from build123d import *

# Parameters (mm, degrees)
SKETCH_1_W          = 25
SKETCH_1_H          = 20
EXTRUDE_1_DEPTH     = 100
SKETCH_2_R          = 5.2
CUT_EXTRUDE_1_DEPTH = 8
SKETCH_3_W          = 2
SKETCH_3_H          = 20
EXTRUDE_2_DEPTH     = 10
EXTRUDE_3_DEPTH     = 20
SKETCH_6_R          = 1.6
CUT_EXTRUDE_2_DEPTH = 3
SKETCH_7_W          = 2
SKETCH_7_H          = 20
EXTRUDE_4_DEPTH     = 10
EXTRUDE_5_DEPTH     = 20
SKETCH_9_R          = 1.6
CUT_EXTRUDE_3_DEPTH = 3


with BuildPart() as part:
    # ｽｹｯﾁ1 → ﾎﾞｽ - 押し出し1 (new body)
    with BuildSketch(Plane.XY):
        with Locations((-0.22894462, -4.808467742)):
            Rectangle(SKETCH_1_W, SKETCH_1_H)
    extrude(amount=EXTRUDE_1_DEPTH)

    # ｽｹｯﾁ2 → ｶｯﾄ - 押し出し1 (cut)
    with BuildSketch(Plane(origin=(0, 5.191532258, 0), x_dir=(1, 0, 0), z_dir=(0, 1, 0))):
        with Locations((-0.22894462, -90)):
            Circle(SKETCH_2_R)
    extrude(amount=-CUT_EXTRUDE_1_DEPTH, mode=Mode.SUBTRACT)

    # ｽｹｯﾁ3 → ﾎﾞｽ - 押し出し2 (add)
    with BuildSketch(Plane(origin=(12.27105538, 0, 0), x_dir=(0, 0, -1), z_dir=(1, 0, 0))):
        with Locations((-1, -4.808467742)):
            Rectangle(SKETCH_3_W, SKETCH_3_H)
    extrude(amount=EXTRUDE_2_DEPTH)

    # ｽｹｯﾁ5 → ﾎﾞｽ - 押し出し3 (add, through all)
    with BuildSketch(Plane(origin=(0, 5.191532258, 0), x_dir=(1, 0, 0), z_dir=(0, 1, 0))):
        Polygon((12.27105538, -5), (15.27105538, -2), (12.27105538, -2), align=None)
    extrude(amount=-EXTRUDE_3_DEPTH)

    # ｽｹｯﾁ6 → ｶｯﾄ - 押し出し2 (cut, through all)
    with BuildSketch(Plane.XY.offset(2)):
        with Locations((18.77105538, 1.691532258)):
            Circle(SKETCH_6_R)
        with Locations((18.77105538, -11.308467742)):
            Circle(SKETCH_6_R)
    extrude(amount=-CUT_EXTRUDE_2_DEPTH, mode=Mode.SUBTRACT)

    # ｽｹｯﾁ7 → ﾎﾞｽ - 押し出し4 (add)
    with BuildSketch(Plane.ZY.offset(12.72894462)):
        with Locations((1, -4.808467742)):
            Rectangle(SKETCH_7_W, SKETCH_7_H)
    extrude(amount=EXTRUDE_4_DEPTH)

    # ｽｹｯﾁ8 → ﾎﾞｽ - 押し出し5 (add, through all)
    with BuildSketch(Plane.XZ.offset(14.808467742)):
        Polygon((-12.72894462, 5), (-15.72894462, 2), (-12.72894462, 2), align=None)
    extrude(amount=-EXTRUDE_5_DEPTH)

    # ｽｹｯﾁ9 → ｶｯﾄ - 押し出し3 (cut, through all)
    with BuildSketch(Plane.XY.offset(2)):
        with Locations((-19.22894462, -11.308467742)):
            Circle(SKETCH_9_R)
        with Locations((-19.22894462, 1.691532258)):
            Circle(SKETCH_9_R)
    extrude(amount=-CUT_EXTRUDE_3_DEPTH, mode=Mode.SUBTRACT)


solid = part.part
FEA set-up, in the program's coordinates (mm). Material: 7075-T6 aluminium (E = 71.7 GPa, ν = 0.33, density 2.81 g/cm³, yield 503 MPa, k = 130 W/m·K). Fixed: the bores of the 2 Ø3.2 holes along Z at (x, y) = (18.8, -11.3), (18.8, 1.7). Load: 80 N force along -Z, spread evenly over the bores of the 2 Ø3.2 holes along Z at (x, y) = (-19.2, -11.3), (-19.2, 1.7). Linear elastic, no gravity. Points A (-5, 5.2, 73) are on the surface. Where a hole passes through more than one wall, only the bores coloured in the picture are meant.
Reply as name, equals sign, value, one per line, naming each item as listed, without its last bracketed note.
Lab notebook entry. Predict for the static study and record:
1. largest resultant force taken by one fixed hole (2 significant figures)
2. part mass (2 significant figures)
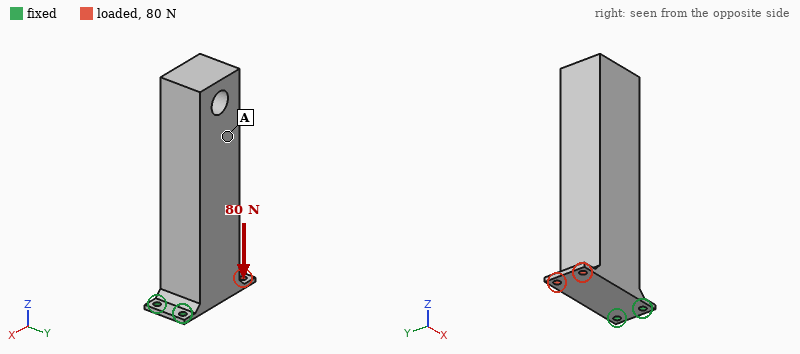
largest resultant force taken by one fixed hole = 41 N
part mass = 140 g
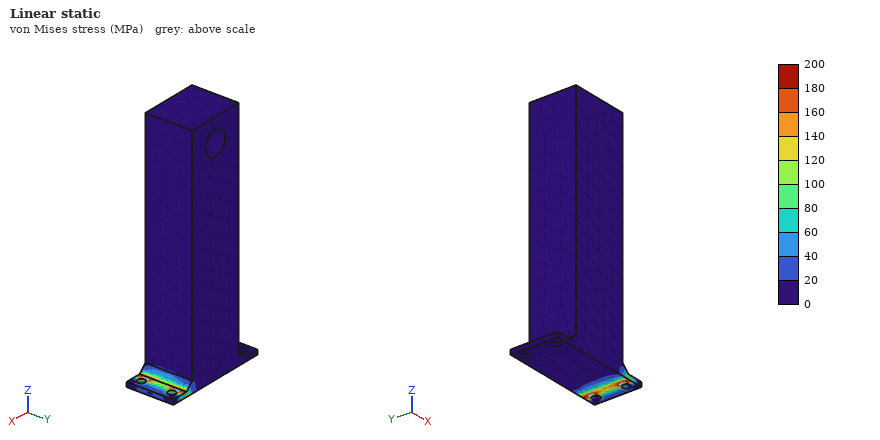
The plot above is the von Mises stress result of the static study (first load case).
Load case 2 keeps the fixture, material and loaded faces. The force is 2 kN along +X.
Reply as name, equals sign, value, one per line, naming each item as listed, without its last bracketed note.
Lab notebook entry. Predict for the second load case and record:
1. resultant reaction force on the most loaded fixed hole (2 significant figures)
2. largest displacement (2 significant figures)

resultant reaction force on the most loaded fixed hole = 1.0 kN
largest displacement = 0.16 mm
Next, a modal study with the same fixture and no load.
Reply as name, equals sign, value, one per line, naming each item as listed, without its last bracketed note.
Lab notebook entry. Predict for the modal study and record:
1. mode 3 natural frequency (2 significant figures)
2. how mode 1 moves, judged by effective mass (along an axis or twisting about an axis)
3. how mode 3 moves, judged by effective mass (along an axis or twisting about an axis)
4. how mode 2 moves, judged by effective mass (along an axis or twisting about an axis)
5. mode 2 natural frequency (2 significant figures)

mode 3 natural frequency = 3000 Hz
how mode 1 moves, judged by effective mass = along X
how mode 3 moves, judged by effective mass = along Z
how mode 2 moves, judged by effective mass = along Y
mode 2 natural frequency = 370 Hz
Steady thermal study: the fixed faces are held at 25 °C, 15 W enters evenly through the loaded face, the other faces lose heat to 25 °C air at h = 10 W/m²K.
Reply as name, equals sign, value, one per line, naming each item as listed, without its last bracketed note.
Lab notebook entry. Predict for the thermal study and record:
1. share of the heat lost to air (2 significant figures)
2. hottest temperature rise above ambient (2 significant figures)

share of the heat lost to air = 14 %
hottest temperature rise above ambient = 52 K
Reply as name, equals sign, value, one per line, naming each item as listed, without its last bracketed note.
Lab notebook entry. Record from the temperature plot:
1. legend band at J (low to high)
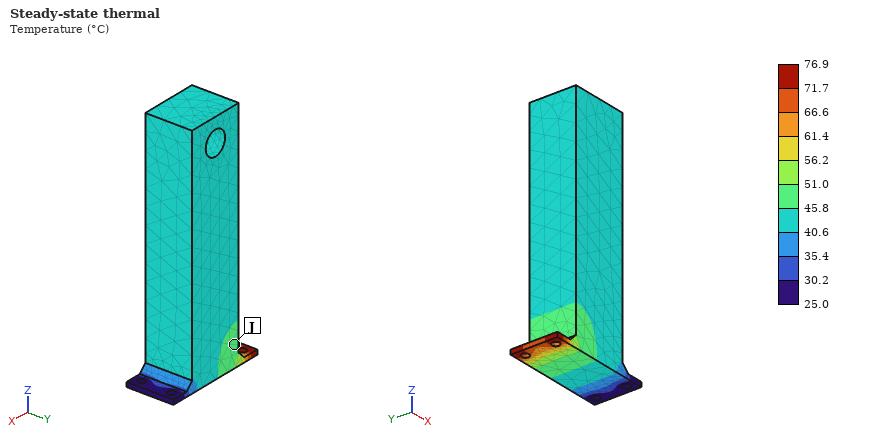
legend band at J = 45.8 to 51.0 °C
